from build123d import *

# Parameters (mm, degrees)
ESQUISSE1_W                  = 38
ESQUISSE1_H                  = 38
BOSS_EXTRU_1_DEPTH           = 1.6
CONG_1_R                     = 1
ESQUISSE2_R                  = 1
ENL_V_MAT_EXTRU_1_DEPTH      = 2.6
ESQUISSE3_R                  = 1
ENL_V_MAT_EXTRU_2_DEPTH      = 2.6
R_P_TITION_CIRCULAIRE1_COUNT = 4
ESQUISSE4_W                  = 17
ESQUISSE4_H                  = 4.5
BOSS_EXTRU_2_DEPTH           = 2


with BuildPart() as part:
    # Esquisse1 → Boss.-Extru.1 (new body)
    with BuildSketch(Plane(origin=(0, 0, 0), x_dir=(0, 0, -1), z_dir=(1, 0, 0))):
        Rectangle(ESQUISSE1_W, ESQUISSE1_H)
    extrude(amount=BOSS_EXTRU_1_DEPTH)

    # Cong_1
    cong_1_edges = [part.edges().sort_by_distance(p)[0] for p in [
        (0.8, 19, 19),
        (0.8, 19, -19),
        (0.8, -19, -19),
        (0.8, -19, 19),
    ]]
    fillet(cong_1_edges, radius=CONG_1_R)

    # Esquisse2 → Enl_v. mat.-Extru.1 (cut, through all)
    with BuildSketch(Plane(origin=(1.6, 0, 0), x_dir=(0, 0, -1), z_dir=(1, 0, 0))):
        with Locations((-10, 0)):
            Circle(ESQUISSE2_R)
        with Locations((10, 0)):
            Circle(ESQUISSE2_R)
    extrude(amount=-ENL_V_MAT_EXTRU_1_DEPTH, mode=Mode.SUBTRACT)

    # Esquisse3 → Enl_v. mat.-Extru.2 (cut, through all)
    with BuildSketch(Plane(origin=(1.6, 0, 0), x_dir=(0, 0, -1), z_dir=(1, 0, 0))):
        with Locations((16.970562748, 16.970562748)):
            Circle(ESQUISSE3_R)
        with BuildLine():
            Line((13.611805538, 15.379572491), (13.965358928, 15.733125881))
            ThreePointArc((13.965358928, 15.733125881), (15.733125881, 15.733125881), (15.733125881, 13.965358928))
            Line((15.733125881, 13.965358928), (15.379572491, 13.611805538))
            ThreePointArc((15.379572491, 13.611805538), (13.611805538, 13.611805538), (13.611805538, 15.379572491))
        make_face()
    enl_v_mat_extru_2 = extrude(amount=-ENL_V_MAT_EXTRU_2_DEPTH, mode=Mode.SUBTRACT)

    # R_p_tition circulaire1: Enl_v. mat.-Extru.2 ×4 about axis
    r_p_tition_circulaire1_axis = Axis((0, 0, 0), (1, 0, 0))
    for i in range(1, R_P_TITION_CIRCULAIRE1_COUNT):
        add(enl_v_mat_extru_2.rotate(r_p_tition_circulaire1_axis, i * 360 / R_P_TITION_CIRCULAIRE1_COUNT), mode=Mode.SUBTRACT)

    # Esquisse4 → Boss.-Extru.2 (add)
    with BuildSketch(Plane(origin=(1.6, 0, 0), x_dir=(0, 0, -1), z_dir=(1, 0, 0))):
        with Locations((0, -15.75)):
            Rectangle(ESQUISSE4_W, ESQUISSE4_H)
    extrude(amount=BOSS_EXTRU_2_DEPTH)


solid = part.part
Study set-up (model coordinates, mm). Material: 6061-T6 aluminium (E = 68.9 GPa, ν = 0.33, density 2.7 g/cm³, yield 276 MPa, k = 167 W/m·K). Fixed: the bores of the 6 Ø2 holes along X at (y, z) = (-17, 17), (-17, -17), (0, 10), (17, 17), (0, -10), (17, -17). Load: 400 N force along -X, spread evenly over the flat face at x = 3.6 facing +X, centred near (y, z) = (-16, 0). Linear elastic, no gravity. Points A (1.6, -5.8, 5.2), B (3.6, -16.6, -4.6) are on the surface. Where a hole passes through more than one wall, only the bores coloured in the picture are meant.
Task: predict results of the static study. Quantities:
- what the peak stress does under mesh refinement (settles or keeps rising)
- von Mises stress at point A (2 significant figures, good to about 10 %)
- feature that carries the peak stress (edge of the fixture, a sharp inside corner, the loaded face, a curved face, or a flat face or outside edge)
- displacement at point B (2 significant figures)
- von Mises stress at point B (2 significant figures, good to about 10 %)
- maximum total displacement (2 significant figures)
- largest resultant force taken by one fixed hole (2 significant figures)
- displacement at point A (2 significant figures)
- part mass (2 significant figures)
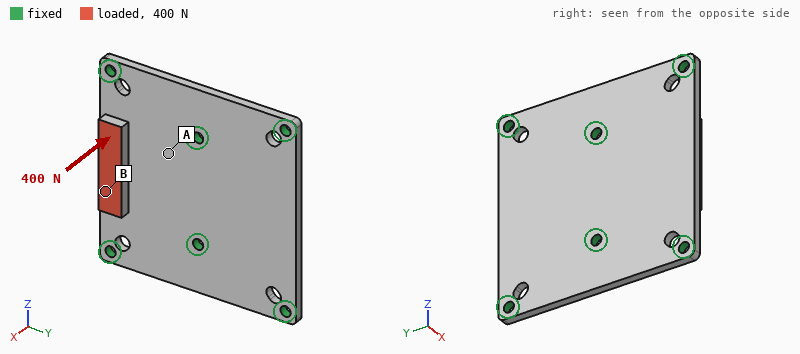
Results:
keeps rising
31 MPa
edge of the fixture
0.11 mm
88 MPa
0.13 mm
220 N
0.028 mm
6.5 g
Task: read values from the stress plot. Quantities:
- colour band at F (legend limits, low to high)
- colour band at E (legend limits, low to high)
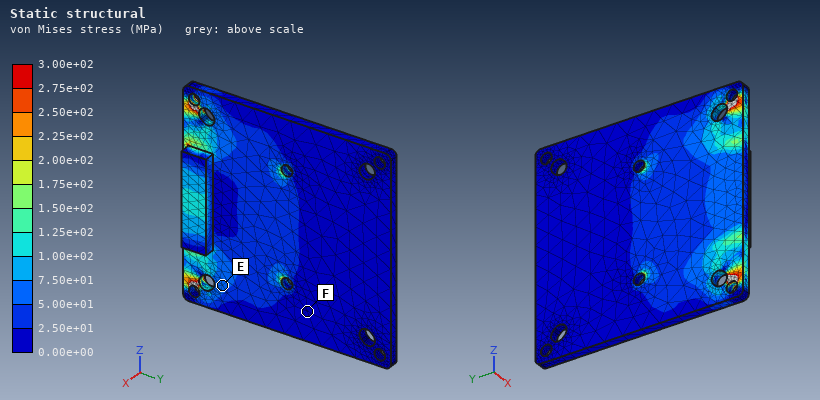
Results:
0.00e+00 to 2.50e+01 MPa
5.00e+01 to 7.50e+01 MPa
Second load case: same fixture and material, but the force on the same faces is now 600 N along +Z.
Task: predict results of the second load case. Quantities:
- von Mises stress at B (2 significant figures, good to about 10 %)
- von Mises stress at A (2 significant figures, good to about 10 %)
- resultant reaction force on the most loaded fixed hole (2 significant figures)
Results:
18 MPa
17 MPa
200 N
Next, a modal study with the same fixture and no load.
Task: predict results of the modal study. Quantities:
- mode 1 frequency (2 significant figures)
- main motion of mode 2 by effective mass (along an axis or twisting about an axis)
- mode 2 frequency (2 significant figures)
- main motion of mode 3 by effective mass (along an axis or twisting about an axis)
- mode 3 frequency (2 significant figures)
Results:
8400 Hz
along X
9200 Hz
along X
18 kHz
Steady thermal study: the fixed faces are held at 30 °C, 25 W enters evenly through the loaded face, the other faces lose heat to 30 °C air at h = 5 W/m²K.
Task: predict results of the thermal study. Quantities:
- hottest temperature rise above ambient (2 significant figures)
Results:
43 K
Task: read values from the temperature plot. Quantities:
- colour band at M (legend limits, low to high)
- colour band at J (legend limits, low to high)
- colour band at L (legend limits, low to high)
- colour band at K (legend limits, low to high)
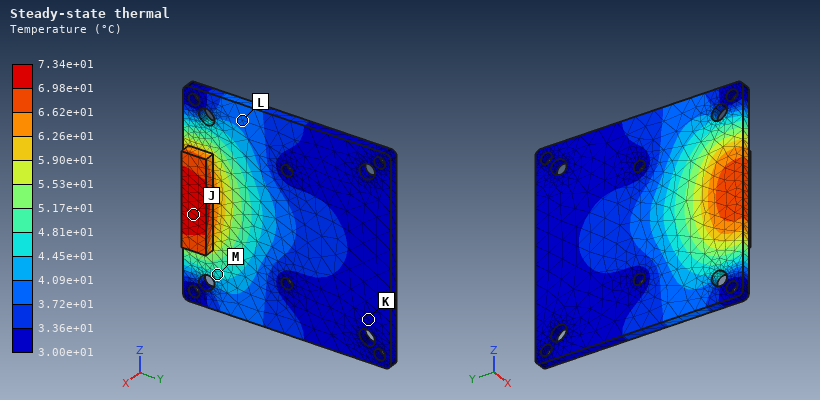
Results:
4.45e+01 to 4.81e+01 °C
6.98e+01 to 7.34e+01 °C
3.72e+01 to 4.09e+01 °C
3.00e+01 to 3.36e+01 °C
